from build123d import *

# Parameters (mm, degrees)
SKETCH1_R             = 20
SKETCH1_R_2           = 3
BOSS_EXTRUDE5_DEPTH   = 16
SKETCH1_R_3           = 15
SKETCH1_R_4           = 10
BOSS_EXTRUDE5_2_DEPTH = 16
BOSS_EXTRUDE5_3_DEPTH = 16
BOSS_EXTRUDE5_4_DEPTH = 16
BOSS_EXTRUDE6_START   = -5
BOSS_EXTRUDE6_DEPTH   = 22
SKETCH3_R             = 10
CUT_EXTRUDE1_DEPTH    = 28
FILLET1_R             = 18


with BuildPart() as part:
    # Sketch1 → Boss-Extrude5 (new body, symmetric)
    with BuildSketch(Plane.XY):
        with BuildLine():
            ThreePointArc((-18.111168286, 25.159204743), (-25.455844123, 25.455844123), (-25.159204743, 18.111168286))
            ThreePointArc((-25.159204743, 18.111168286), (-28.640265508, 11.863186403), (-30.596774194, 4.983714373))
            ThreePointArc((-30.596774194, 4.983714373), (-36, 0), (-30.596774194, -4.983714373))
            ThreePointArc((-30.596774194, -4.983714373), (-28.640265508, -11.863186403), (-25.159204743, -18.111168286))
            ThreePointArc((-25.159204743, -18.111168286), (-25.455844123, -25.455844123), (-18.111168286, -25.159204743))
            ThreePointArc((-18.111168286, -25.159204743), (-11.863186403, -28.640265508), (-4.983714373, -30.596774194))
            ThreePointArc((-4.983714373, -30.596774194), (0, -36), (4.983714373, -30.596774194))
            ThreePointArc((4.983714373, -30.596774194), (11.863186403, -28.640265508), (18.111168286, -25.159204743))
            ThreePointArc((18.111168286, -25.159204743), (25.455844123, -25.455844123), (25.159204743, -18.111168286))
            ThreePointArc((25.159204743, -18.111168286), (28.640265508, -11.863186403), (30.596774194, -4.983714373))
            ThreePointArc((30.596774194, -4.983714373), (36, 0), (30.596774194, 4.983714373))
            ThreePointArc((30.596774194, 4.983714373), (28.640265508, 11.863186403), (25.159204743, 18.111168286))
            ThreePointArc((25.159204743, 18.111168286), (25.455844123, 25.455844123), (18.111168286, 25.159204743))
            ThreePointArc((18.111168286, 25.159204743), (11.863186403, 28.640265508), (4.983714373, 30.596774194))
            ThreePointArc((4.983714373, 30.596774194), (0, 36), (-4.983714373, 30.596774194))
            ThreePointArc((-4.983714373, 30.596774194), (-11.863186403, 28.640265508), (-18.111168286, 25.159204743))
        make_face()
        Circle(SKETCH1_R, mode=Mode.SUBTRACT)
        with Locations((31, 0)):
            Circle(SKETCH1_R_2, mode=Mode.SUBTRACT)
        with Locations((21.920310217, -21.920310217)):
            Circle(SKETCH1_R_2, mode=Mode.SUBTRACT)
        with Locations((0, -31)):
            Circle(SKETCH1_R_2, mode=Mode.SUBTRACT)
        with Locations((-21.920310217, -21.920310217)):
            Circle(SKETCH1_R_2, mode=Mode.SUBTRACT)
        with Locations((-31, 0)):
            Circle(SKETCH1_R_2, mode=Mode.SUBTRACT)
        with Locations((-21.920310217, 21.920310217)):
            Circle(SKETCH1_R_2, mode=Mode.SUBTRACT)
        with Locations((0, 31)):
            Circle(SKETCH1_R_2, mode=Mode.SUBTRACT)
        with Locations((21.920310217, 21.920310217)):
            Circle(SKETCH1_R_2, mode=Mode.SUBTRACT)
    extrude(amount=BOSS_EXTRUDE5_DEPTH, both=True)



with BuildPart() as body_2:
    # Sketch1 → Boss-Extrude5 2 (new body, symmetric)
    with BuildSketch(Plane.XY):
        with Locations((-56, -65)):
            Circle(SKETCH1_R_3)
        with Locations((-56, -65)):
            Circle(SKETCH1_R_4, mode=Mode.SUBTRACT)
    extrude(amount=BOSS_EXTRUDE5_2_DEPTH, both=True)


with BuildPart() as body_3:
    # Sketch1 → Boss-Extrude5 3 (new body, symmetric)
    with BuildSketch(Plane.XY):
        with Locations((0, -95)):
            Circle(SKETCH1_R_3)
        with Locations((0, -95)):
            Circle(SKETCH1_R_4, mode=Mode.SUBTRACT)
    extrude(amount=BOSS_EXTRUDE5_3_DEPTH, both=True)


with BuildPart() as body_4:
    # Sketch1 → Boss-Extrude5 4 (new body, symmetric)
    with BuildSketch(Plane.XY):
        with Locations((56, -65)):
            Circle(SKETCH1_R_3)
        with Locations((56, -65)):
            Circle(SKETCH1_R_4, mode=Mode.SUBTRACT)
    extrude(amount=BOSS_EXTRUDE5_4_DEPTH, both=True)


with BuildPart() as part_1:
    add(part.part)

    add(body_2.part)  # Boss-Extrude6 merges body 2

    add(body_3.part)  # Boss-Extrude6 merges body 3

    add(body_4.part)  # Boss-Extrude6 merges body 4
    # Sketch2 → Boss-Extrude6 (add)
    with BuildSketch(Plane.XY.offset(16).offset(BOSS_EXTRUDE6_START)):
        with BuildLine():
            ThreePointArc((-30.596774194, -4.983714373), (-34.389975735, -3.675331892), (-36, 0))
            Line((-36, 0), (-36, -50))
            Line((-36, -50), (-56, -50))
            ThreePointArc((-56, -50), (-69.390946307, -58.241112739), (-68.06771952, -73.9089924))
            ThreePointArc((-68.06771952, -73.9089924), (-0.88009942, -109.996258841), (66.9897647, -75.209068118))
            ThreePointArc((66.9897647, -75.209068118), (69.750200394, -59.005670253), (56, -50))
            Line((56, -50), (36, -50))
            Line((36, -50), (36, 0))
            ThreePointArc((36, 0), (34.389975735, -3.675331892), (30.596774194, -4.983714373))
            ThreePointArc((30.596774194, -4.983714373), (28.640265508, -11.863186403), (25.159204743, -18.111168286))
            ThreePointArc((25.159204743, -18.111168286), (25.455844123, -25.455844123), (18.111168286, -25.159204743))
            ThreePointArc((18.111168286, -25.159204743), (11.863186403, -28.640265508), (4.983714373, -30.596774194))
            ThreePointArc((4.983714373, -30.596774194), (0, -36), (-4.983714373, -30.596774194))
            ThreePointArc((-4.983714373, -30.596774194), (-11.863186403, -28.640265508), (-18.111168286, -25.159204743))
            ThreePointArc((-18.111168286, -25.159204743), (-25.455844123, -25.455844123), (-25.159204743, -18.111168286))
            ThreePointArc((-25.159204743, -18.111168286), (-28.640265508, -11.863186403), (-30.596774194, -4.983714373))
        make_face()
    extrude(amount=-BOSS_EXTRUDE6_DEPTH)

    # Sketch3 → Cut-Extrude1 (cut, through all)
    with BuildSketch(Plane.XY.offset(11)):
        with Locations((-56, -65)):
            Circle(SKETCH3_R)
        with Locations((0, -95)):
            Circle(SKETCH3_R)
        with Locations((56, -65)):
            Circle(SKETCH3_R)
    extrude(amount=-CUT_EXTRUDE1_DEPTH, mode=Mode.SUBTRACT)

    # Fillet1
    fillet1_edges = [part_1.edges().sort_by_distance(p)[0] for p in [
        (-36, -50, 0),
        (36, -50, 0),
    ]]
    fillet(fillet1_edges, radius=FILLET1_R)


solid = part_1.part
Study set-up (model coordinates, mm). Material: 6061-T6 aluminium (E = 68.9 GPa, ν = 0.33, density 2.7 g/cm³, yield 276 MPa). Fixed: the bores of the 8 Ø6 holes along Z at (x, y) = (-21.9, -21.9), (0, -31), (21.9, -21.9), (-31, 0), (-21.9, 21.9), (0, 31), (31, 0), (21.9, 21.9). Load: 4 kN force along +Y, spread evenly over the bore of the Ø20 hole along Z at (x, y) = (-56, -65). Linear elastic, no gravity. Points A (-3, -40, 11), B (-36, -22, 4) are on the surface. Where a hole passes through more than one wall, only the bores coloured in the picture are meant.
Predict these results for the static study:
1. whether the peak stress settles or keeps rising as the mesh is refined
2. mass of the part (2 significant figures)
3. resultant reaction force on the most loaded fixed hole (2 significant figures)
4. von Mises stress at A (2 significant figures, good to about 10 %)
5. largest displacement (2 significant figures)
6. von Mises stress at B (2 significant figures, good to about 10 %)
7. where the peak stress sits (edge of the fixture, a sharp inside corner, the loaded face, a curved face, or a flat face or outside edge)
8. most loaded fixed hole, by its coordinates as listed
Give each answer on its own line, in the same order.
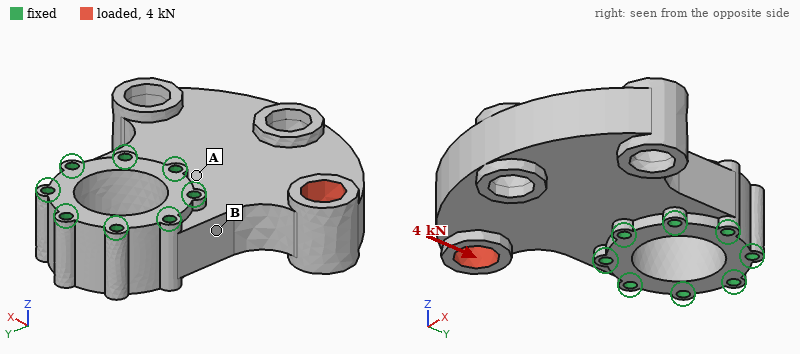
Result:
keeps rising
660 g
4.7 kN
3.2 MPa
29 µm
8.8 MPa
edge of the fixture
(-21.9, -21.9)
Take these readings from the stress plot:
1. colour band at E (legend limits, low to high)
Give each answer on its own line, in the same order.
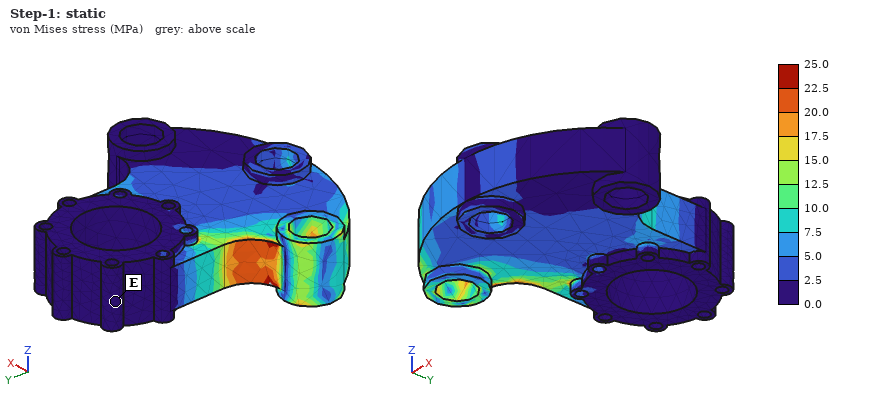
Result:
0.0 to 2.5 MPa
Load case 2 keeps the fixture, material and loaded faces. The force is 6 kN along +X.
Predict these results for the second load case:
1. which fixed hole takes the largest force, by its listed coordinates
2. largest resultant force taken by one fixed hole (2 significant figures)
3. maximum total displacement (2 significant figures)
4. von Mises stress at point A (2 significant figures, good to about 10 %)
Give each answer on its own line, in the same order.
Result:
(0, -31)
4.4 kN
21 µm
11 MPa
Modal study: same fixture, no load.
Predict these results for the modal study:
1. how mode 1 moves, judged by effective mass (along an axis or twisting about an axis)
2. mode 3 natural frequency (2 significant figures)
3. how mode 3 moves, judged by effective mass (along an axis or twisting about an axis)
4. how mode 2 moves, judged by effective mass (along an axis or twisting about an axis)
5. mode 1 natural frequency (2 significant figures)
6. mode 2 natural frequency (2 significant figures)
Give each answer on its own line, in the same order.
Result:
along Z
4300 Hz
along X
twisting about Y
2400 Hz
3200 Hz
